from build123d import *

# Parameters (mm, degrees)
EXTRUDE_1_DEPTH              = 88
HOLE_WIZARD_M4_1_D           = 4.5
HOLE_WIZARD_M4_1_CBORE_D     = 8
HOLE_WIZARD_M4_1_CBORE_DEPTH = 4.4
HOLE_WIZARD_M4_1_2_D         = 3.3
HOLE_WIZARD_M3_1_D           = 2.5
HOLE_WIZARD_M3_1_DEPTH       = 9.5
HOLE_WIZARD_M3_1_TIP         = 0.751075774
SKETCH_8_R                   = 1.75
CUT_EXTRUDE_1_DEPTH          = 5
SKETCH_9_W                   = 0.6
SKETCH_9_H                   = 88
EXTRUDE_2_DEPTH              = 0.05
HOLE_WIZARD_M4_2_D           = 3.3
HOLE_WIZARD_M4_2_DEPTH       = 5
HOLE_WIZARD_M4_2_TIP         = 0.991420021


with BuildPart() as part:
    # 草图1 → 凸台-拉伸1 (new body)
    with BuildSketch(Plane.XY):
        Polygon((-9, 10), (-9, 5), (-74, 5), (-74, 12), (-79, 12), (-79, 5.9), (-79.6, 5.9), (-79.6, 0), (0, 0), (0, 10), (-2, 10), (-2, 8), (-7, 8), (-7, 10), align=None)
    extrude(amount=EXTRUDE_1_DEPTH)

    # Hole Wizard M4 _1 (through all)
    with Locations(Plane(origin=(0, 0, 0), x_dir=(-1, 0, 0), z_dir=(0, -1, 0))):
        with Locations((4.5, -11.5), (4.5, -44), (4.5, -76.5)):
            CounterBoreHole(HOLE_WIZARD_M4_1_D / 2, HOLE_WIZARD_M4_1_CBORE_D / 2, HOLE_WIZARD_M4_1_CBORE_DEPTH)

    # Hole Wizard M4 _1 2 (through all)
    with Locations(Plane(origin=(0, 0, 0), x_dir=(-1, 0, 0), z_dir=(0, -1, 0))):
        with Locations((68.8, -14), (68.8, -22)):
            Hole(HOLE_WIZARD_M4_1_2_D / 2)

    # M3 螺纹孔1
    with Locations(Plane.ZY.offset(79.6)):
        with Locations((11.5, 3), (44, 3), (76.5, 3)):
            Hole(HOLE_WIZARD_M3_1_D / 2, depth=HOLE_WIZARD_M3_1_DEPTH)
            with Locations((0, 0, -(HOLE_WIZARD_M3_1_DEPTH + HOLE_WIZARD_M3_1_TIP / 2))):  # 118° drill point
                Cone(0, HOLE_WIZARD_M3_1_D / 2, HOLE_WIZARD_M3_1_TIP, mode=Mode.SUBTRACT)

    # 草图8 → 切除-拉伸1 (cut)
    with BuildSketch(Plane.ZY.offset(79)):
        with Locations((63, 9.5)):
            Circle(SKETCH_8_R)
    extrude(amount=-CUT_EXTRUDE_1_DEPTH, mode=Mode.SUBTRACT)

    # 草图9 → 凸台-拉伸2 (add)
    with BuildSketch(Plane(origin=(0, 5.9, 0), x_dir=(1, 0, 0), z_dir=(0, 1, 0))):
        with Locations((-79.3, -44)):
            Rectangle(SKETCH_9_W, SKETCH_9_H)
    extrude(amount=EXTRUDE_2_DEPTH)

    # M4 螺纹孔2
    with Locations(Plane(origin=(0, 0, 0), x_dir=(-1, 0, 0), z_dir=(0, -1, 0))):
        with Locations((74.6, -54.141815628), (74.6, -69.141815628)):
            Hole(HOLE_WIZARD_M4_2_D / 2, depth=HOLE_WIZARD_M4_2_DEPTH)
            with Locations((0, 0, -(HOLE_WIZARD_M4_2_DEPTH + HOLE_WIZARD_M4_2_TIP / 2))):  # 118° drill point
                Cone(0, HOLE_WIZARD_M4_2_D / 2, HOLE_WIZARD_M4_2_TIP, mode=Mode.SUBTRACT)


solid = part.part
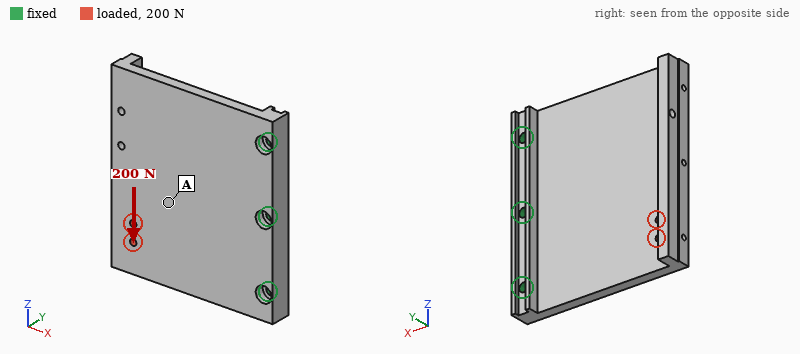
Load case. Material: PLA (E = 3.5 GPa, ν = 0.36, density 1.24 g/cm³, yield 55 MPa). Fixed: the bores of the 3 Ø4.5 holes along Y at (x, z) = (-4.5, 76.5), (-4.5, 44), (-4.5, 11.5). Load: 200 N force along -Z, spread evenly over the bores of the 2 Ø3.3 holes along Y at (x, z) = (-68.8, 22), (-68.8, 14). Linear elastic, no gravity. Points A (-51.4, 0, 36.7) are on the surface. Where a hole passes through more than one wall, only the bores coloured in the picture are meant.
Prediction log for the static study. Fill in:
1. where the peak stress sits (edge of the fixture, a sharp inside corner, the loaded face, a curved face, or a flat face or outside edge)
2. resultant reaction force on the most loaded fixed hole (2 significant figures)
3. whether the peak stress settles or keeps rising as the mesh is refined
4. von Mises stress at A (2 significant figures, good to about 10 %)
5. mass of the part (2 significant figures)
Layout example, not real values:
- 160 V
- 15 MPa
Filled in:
- edge of the fixture
- 200 N
- keeps rising
- 1.1 MPa
- 50 g
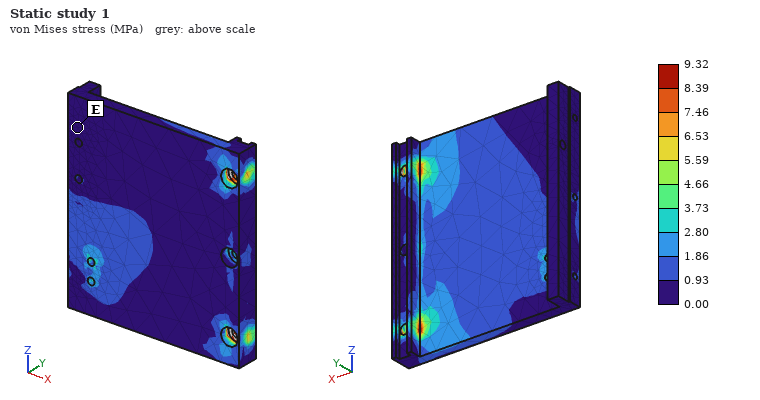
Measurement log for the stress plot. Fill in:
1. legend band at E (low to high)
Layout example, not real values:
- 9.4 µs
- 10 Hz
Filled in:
- 0.00 to 0.93 MPa
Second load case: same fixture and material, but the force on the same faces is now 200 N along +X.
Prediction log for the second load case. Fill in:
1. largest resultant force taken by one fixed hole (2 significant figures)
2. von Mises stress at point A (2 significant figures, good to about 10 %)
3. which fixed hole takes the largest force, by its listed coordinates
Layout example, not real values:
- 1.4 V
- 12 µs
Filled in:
- 140 N
- 0.57 MPa
- (-4.5, 11.5)
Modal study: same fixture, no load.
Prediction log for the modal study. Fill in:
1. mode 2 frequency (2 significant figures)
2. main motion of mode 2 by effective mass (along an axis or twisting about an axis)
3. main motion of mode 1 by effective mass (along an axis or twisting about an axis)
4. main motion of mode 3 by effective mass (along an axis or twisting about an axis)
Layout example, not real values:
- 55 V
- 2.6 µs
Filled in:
- 450 Hz
- twisting about X
- along Y
- along Y
